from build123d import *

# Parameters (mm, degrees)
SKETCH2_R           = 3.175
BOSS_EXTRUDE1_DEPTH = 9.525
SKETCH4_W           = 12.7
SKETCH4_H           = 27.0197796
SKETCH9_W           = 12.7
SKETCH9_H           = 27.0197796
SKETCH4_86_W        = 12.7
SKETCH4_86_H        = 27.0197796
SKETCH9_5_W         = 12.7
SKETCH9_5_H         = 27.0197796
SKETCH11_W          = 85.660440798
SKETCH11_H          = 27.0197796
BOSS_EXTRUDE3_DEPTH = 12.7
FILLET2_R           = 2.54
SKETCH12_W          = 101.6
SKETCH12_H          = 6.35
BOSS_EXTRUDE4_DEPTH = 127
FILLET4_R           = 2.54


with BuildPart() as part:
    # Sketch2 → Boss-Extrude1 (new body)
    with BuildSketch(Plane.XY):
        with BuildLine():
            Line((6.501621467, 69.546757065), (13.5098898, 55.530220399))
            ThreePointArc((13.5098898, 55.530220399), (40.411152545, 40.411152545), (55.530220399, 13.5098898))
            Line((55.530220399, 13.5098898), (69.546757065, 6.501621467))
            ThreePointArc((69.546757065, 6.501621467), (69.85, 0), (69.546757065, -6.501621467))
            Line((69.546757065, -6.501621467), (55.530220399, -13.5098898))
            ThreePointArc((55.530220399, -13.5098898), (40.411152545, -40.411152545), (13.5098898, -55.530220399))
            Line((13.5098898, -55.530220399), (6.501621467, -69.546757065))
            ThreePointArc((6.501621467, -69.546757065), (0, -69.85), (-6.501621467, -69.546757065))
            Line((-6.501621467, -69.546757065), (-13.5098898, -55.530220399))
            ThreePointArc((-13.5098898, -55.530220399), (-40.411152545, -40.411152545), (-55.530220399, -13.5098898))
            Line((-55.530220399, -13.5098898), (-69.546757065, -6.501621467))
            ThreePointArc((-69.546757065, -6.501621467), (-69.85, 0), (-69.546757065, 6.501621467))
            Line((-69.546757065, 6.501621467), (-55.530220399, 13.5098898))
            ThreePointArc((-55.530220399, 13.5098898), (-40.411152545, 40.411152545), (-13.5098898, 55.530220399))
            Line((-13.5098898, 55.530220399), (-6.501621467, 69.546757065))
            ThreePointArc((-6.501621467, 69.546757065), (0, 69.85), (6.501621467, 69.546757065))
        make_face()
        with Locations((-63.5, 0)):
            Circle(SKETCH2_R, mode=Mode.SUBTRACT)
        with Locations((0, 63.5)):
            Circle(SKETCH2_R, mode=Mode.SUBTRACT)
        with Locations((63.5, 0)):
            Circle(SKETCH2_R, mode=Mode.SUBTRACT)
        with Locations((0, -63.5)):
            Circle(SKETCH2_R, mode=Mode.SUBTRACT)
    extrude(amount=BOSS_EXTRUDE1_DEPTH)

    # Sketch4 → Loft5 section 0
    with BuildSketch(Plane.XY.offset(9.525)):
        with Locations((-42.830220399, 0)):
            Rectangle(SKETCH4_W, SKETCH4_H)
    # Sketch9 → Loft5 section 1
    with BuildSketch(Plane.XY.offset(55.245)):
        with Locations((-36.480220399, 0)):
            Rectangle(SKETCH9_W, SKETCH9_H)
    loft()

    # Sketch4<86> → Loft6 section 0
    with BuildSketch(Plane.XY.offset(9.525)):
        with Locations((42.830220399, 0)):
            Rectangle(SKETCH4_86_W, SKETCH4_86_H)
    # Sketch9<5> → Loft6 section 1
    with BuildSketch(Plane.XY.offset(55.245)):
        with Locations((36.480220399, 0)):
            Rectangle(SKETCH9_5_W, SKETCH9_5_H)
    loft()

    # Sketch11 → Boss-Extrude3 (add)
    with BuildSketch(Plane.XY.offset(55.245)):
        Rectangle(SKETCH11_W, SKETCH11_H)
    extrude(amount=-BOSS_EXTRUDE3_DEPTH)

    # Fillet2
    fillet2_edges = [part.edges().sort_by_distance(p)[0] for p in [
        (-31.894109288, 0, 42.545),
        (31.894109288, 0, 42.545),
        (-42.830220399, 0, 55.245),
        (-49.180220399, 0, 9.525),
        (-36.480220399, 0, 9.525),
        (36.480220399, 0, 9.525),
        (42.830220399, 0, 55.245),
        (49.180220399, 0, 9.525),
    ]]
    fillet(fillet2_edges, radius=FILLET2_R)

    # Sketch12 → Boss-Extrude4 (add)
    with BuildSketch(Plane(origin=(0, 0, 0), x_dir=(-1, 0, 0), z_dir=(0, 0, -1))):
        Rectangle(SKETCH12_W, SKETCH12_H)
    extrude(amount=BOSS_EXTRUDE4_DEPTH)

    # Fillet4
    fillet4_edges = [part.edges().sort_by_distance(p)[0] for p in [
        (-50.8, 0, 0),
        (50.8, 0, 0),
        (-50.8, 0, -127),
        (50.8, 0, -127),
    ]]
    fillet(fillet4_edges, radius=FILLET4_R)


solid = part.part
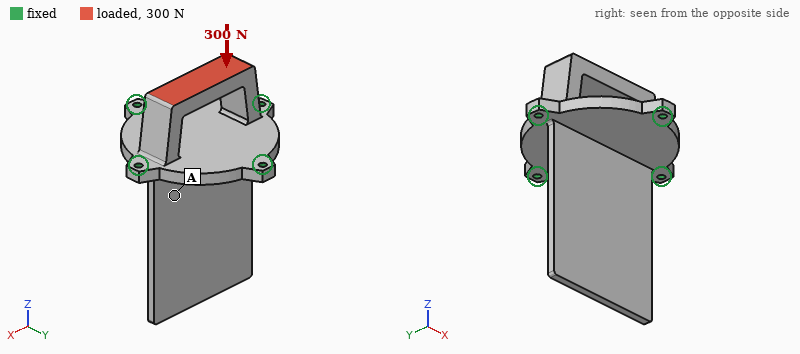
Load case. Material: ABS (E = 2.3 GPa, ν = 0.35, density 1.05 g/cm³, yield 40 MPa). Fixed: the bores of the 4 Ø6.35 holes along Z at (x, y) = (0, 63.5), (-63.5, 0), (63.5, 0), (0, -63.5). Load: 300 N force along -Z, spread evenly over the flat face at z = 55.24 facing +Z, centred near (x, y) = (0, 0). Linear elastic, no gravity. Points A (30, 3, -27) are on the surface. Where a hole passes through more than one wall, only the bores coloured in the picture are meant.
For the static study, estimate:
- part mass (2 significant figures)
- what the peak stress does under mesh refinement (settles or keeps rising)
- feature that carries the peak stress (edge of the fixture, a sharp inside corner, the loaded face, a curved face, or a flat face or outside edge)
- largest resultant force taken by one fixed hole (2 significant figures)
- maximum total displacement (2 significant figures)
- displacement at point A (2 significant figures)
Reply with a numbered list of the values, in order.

1. 250 g
2. keeps rising
3. edge of the fixture
4. 140 N
5. 84 µm
6. 23 µm
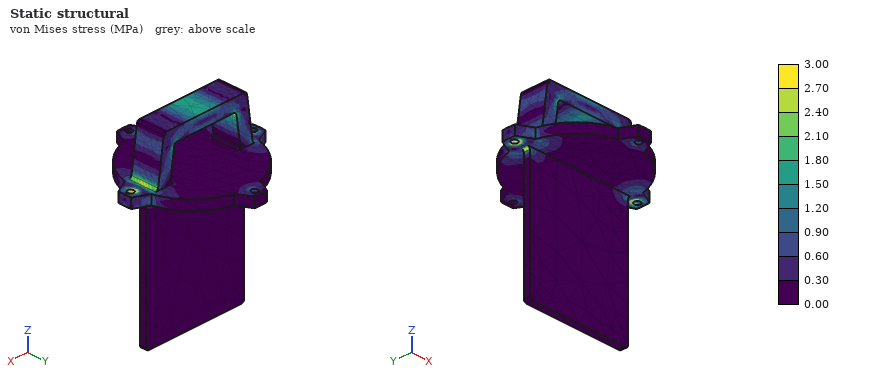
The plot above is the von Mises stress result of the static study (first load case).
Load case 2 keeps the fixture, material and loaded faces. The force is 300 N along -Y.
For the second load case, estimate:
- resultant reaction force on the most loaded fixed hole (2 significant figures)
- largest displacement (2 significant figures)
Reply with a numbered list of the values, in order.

1. 140 N
2. 0.56 mm
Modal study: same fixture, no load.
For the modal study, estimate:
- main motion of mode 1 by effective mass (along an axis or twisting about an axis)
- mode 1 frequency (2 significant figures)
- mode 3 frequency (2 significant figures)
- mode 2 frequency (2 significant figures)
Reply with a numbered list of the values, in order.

1. along Y
2. 92 Hz
3. 550 Hz
4. 270 Hz
